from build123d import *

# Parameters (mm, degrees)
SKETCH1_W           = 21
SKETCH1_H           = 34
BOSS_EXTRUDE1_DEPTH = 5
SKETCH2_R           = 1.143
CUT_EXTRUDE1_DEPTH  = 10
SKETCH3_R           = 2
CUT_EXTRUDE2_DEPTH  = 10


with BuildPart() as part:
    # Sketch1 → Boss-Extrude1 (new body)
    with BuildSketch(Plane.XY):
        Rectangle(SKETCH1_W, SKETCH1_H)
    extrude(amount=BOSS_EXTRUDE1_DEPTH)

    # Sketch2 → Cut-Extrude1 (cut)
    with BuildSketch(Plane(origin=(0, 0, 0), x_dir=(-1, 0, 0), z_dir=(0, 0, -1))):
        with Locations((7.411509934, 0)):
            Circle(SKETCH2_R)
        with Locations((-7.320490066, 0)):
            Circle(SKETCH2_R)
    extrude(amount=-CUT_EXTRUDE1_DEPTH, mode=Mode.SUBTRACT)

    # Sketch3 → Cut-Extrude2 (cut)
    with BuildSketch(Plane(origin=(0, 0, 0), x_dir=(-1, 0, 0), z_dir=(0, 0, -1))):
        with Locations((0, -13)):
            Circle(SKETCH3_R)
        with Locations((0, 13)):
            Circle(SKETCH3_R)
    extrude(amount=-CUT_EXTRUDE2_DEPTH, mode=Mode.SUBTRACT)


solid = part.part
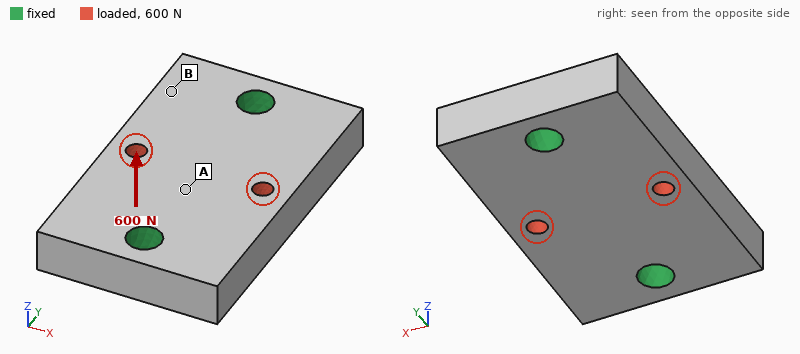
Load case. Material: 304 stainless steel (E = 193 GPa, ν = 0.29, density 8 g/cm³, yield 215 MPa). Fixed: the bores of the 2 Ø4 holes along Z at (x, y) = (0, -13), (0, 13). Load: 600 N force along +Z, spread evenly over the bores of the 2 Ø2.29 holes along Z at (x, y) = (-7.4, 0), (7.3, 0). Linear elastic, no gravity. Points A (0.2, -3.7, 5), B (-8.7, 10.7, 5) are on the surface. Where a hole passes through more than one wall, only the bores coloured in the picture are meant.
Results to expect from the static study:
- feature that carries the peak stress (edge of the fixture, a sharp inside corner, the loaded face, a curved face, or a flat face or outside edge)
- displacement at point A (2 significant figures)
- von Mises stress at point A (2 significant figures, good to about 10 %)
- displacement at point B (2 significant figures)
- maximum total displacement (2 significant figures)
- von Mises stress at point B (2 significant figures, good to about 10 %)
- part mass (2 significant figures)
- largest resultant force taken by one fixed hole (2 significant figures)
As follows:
the loaded face
1.6 µm
18 MPa
1.1 µm
3.4 µm
6.1 MPa
27 g
300 N
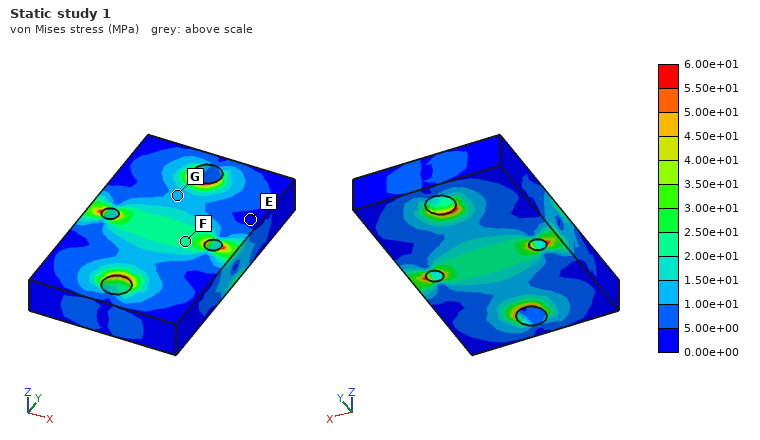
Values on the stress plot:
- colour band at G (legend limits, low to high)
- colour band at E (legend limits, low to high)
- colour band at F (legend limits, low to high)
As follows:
1.00e+01 to 1.50e+01 MPa
0.00e+00 to 5.00e+00 MPa
2.00e+01 to 2.50e+01 MPa
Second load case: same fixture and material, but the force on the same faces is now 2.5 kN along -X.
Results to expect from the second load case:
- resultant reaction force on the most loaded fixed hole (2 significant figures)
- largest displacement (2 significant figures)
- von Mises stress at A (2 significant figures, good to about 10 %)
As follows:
1.3 kN
3.7 µm
23 MPa
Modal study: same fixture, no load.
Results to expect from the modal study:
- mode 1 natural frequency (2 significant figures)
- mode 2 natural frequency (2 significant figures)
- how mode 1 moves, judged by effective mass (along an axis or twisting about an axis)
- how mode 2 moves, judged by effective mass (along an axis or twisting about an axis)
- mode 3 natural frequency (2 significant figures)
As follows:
23 kHz
26 kHz
twisting about Y
along Z
39 kHz
